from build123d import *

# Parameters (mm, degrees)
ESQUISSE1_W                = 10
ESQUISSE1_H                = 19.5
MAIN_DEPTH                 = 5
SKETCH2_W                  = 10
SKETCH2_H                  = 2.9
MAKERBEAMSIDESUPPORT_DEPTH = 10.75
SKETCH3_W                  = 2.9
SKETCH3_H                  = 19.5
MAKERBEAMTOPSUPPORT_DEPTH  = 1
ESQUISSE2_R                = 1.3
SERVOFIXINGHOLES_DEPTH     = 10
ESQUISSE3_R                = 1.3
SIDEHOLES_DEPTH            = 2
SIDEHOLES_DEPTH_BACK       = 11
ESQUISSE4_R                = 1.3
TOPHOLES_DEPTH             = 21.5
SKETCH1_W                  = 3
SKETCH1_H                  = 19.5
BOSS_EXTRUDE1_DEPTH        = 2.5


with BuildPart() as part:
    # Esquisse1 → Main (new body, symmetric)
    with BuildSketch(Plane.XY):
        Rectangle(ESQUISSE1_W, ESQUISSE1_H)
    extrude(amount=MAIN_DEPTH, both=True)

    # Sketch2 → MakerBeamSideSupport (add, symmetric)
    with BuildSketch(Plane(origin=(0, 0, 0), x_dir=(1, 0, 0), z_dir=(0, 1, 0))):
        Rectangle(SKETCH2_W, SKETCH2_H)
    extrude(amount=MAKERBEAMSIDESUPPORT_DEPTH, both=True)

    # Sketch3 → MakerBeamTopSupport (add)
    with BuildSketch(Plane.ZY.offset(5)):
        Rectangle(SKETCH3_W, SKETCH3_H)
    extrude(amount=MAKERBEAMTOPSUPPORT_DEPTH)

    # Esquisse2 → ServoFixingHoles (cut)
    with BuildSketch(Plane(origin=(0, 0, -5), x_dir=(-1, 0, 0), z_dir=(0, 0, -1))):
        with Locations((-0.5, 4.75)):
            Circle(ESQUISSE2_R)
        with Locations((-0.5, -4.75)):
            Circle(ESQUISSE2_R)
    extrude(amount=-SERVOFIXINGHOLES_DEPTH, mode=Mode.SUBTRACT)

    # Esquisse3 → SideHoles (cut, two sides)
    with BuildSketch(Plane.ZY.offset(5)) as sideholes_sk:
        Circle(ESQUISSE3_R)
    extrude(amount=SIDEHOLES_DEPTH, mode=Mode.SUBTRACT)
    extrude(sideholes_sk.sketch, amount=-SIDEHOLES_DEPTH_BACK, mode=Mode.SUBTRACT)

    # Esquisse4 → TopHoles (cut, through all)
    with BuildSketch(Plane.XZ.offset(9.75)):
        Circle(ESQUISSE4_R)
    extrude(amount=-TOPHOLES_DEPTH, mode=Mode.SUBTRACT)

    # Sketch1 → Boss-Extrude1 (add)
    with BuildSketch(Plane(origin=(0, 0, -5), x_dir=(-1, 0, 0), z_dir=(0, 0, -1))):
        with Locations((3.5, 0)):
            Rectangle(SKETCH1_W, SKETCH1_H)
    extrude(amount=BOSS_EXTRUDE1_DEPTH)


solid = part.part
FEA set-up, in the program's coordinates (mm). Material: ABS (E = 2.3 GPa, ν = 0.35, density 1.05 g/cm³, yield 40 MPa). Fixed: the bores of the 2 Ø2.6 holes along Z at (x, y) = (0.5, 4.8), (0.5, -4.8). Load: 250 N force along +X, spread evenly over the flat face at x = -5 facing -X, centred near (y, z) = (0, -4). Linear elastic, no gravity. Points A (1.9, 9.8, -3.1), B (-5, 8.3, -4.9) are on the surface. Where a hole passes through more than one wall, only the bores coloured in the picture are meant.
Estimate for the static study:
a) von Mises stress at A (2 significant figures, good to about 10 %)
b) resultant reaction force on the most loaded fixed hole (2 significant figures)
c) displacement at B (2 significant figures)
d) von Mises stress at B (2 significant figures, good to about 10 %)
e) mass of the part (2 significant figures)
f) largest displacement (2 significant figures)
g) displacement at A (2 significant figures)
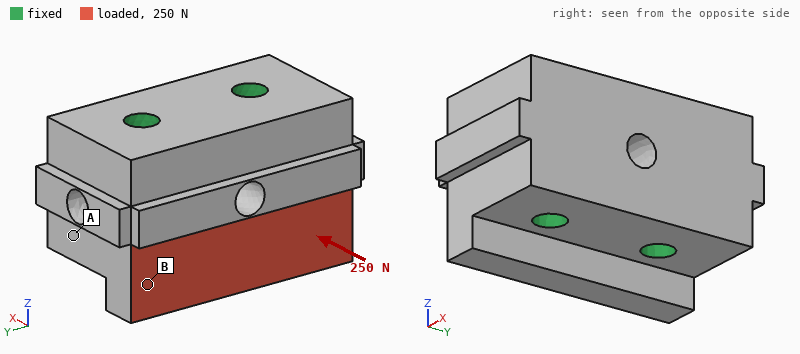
1.5 MPa
130 N
20 µm
4.5 MPa
2.1 g
33 µm
5.5 µm
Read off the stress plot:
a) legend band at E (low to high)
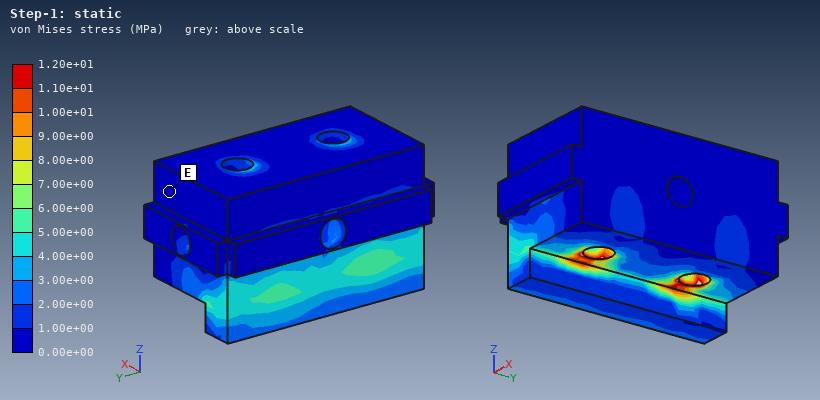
0.00e+00 to 1.00e+00 MPa
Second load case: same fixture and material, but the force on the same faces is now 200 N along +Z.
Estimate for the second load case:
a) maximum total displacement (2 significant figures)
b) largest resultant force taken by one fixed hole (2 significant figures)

38 µm
100 N
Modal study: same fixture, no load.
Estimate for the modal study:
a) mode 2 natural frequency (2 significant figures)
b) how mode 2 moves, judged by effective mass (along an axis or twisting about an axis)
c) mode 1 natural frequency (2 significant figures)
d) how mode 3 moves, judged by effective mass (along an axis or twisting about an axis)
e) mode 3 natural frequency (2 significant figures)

23 kHz
along Z
22 kHz
twisting about X
25 kHz
